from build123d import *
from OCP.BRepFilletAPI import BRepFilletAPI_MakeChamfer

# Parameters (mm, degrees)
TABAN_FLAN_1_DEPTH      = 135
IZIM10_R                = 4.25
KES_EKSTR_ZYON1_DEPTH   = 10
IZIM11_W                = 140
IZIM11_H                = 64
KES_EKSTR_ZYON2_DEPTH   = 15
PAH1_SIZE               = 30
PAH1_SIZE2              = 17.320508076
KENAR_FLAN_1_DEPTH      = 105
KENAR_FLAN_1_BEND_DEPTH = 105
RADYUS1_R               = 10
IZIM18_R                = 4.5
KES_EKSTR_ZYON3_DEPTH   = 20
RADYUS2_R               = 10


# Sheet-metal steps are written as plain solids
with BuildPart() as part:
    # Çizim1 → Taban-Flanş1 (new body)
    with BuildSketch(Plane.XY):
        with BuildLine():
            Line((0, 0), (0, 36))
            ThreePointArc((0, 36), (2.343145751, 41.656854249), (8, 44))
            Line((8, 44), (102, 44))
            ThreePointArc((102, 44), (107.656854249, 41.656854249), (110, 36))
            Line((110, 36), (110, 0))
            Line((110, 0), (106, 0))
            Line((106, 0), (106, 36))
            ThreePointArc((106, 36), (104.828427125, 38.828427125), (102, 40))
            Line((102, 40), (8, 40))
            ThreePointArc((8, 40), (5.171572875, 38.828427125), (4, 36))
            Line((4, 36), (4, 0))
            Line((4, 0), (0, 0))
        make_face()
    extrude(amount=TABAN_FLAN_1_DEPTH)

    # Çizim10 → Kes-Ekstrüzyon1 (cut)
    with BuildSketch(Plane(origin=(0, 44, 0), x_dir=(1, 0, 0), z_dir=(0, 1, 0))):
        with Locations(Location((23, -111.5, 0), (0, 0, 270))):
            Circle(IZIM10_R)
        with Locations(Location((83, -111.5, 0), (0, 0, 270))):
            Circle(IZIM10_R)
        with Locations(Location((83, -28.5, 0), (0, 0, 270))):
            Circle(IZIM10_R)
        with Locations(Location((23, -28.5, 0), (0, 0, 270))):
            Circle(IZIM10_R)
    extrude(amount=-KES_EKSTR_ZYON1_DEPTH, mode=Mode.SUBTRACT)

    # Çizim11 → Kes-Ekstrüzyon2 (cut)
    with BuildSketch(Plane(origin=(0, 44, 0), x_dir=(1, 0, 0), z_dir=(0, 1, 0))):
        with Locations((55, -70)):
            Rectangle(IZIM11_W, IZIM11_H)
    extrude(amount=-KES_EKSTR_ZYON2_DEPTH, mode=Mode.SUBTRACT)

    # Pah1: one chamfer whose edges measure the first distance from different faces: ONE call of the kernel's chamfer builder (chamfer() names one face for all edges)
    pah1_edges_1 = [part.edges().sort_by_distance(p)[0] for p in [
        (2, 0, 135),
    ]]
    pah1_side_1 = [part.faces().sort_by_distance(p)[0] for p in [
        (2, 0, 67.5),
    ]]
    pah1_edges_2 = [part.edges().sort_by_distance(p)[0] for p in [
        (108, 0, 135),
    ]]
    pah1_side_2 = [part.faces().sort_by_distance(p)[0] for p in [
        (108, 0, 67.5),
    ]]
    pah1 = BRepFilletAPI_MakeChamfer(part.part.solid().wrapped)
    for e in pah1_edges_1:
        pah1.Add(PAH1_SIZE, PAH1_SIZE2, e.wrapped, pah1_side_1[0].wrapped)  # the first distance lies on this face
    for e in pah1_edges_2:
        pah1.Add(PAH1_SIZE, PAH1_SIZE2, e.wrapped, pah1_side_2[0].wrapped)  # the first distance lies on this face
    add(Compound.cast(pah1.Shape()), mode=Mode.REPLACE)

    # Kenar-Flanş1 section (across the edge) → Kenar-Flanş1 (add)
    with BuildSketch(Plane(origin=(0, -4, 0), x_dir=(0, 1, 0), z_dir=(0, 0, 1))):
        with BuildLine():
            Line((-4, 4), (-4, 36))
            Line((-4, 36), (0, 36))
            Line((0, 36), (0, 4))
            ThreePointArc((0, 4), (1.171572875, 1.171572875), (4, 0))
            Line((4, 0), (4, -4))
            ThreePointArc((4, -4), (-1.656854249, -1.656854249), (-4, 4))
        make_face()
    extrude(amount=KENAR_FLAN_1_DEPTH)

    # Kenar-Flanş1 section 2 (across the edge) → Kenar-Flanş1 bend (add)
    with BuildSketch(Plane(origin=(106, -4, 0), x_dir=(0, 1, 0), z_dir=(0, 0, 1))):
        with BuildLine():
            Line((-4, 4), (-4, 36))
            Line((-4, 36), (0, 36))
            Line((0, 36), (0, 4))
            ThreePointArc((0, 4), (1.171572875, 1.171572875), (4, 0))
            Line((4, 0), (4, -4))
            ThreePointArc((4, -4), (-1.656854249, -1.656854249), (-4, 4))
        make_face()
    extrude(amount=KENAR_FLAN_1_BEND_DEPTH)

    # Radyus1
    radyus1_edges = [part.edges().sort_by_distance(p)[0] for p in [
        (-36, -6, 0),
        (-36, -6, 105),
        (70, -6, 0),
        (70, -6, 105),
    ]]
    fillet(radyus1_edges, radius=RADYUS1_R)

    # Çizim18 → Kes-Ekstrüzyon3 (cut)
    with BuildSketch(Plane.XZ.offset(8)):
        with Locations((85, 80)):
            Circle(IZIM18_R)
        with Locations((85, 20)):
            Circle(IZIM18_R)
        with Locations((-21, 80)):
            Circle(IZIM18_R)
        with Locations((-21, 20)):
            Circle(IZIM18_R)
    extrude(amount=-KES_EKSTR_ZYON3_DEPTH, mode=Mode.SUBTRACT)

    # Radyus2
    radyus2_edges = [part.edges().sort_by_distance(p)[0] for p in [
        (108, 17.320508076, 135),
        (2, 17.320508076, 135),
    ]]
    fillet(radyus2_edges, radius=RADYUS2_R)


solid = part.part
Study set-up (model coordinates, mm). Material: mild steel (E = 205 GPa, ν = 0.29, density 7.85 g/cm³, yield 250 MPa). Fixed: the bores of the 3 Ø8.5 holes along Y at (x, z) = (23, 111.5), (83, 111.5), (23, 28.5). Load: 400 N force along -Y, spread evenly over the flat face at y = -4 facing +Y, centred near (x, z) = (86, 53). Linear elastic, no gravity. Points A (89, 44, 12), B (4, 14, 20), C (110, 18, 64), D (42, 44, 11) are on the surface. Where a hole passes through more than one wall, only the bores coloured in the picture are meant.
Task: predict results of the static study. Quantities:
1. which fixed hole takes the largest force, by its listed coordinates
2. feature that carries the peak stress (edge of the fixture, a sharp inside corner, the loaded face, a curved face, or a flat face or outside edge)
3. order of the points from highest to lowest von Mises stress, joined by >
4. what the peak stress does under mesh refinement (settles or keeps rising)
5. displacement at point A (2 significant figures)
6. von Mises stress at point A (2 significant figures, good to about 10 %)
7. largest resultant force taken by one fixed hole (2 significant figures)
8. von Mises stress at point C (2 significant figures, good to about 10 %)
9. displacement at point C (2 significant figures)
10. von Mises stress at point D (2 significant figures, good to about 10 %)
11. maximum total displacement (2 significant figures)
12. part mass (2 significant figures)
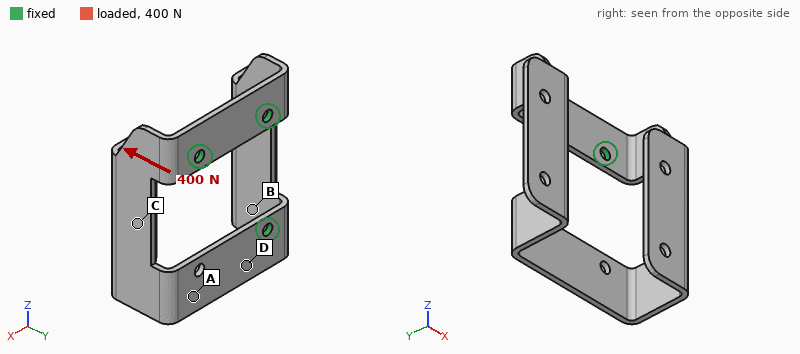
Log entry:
(83, 111.5)
edge of the fixture
D > A > C > B
keeps rising
0.24 mm
31 MPa
220 N
16 MPa
0.16 mm
44 MPa
0.48 mm
770 g
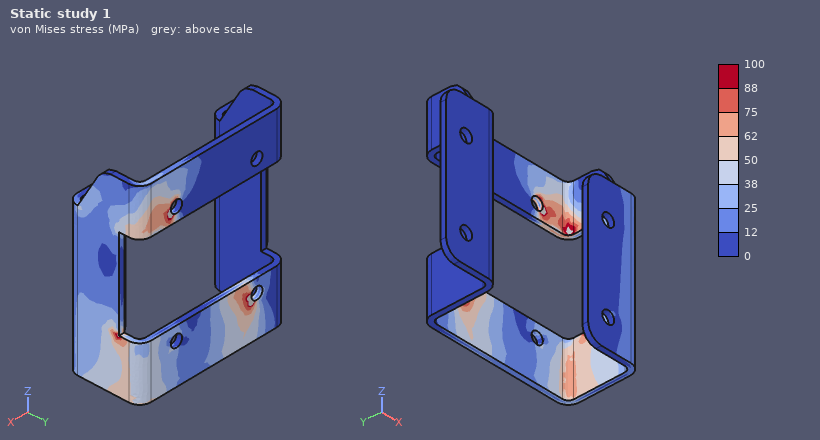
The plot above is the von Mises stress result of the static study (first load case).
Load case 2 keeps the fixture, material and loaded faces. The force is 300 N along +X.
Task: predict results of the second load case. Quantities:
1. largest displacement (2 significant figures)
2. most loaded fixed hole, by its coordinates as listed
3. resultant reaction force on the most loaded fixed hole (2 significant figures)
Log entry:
0.57 mm
(23, 28.5)
200 N
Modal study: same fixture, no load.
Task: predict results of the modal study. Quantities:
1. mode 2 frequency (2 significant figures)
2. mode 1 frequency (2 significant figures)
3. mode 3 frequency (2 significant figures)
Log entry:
350 Hz
250 Hz
380 Hz
